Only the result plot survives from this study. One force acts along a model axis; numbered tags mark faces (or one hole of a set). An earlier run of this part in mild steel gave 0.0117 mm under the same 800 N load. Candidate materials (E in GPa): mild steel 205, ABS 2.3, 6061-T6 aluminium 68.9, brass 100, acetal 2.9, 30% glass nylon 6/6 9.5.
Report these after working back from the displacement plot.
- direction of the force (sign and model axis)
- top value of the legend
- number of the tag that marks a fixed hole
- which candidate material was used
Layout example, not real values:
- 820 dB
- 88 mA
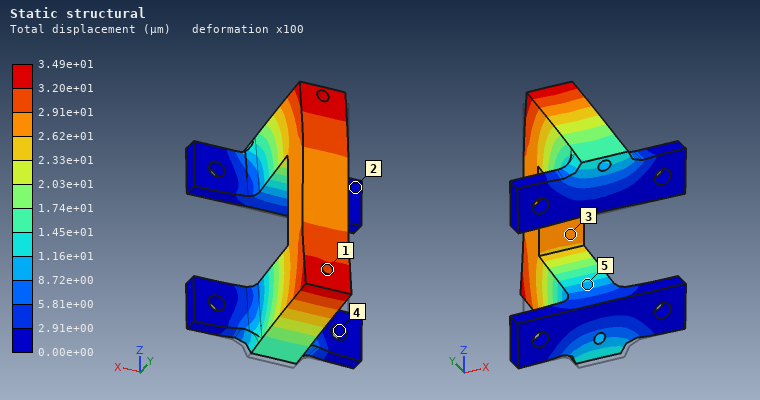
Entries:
- +Z
- 3.49e+01 µm
- 4
- 6061-T6 aluminium
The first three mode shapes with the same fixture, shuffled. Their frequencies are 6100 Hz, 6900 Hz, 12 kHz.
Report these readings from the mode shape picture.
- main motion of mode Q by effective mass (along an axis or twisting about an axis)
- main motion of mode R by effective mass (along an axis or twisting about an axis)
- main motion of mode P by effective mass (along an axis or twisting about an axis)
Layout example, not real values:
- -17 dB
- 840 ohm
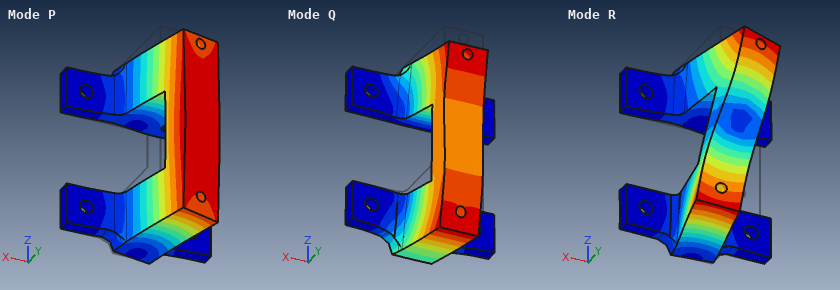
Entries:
- along Z
- twisting about Y
- along X
